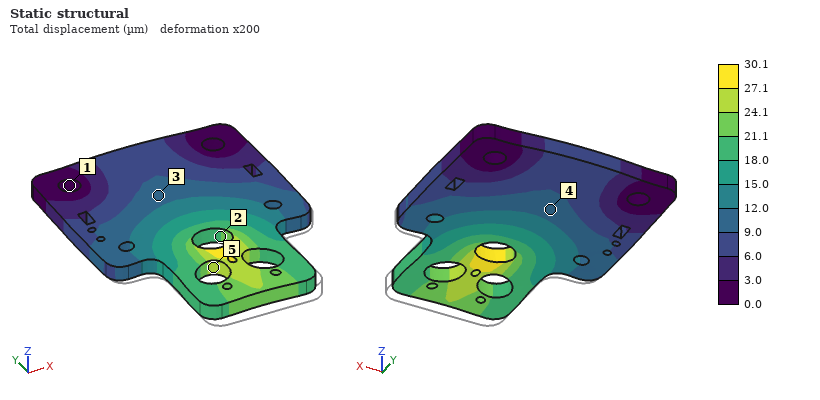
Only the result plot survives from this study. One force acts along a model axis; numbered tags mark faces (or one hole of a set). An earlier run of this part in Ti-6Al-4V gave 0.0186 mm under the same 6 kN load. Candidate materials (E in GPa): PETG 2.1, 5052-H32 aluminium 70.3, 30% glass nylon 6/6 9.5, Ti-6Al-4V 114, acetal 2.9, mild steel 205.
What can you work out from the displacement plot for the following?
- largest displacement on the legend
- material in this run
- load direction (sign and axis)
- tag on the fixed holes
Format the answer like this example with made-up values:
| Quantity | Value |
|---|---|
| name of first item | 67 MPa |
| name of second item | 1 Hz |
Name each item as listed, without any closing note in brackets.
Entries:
| Quantity | Value |
|---|---|
| largest displacement on the legend | 30.1 µm |
| material in this run | 5052-H32 aluminium |
| load direction | +Y |
| tag on the fixed holes | 1 |
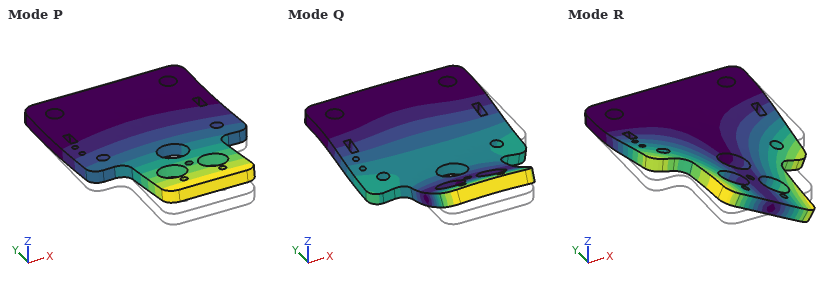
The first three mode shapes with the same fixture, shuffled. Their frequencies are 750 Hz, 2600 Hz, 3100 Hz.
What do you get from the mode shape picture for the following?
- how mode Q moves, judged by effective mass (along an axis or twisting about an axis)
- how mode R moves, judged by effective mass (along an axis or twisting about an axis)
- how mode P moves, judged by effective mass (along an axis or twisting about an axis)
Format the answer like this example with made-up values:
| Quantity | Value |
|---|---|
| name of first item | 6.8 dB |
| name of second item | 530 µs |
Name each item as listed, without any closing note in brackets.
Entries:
| Quantity | Value |
|---|---|
| how mode Q moves, judged by effective mass | along Z |
| how mode R moves, judged by effective mass | twisting about Y |
| how mode P moves, judged by effective mass | along Z |
